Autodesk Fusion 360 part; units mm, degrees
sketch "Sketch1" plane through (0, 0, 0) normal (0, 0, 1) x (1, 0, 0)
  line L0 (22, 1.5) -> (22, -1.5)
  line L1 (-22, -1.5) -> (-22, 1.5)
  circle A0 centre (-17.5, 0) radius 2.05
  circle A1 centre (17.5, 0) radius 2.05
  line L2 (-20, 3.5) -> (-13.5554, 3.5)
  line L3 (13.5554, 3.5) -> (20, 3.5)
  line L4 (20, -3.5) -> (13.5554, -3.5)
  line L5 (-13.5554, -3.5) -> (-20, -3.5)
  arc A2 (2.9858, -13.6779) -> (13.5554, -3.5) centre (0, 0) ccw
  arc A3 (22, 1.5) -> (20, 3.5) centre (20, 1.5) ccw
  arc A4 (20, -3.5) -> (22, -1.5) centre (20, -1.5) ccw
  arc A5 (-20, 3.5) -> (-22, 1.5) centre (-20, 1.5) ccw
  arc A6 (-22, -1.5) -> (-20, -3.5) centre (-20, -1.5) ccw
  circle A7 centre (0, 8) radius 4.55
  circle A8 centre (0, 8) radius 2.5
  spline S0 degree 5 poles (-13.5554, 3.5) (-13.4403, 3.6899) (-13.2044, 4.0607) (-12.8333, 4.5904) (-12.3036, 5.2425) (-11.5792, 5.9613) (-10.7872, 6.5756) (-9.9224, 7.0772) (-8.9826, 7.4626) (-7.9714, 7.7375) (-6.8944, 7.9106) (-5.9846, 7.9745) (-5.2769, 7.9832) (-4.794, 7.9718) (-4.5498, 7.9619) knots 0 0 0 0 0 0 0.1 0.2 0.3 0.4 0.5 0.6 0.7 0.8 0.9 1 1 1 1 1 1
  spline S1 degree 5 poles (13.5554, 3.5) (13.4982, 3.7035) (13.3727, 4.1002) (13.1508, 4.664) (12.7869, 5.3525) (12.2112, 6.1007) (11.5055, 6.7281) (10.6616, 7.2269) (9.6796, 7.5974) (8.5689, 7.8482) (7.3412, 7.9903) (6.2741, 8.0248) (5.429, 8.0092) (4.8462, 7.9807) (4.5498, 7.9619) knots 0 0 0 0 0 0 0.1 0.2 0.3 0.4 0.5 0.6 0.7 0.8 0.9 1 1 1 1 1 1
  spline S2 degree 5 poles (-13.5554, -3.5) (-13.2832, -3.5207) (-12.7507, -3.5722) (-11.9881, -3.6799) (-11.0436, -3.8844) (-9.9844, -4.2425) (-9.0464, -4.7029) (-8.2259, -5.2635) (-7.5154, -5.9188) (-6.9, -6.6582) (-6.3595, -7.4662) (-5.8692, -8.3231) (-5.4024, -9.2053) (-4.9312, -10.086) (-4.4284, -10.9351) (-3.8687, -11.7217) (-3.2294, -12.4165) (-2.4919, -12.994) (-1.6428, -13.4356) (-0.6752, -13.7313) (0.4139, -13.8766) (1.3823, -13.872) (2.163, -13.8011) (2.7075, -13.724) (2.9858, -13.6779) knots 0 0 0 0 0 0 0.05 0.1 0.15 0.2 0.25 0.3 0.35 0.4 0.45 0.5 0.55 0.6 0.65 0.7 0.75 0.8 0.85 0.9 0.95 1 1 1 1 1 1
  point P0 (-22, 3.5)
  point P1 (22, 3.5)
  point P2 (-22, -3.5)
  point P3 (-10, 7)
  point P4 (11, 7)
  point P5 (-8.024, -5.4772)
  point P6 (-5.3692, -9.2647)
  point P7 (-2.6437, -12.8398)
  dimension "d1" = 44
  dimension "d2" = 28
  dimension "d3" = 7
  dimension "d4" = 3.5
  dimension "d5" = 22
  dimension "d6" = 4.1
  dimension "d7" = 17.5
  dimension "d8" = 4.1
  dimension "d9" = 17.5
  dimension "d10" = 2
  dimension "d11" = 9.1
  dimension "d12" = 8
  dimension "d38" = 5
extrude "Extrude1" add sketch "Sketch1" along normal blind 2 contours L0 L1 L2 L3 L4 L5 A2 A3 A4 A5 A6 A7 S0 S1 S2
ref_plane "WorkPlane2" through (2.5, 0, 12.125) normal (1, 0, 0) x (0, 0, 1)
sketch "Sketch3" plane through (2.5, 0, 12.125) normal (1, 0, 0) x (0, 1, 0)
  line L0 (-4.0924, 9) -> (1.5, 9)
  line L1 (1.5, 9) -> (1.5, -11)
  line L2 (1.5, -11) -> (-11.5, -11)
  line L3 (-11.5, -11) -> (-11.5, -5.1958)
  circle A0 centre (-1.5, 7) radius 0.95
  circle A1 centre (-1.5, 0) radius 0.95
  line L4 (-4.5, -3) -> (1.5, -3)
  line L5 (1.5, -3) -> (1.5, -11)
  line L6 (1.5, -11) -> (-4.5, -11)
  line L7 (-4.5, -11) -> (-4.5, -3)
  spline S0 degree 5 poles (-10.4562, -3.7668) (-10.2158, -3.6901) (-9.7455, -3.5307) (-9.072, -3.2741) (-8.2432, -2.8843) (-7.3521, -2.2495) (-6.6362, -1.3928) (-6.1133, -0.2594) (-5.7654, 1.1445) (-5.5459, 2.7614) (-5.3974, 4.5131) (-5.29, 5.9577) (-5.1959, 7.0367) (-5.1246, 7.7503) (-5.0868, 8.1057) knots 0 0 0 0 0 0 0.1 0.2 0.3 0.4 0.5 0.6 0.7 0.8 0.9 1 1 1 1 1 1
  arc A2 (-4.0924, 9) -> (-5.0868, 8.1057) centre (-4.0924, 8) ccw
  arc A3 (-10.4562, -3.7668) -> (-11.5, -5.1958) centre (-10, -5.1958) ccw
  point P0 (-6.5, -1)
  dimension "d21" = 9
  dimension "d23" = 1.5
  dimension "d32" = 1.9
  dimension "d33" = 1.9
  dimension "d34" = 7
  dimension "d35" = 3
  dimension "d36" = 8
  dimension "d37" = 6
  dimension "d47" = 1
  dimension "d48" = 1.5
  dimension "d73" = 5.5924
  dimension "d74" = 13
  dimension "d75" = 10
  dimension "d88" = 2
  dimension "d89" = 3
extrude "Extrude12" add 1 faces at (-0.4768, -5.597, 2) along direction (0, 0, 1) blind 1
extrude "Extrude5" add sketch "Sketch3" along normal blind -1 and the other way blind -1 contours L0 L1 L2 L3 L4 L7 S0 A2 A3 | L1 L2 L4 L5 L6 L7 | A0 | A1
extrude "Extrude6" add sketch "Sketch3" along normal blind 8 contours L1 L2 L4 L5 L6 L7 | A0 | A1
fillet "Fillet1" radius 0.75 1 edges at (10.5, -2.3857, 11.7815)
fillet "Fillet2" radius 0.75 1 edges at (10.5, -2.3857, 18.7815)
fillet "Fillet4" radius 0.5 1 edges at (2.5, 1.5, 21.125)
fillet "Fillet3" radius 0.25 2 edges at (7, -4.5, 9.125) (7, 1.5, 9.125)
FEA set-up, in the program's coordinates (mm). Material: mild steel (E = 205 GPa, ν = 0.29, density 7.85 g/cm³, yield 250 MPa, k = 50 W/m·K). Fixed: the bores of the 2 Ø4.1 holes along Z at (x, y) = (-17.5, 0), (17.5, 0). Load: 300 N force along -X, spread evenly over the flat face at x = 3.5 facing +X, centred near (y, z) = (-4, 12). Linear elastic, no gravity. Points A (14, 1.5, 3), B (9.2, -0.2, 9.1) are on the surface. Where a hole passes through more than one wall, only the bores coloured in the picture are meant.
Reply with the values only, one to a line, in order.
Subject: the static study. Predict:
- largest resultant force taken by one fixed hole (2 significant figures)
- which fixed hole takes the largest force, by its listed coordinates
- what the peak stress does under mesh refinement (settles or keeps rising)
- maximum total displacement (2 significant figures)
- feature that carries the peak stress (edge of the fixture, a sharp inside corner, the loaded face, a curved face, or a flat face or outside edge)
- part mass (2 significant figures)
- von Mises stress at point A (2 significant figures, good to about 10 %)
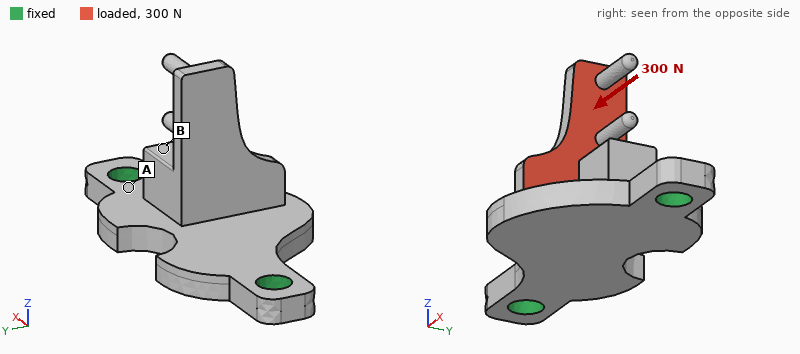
230 N
(17.5, 0)
keeps rising
76 µm
a sharp inside corner
17 g
33 MPa
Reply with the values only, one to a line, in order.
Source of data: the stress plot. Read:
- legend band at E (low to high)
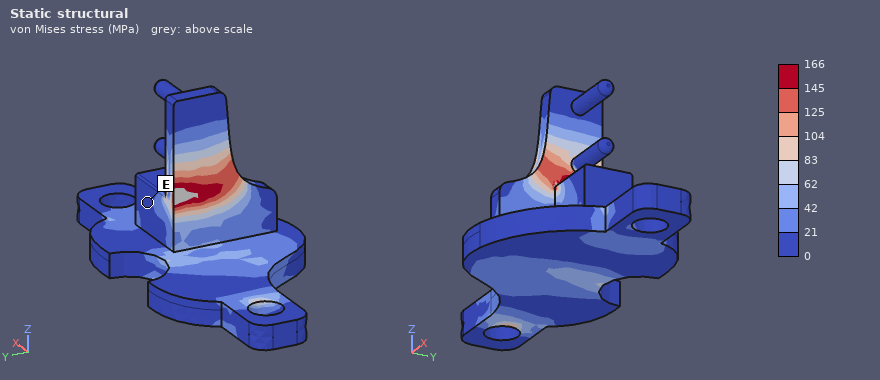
0 to 21 MPa
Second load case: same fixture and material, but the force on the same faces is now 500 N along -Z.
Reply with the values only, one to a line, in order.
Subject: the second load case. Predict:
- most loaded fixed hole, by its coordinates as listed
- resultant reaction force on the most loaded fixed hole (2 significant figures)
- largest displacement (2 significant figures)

(17.5, 0)
320 N
38 µm
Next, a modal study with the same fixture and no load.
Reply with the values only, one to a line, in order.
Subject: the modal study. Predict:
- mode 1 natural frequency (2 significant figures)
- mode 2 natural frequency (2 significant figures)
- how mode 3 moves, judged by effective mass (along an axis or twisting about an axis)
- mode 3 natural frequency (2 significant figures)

5900 Hz
7300 Hz
along Z
10 kHz
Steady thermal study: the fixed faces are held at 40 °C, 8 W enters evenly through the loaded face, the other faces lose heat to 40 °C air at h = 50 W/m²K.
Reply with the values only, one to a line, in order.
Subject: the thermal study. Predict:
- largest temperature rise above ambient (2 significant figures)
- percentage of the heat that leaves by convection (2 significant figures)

77 K
27 %
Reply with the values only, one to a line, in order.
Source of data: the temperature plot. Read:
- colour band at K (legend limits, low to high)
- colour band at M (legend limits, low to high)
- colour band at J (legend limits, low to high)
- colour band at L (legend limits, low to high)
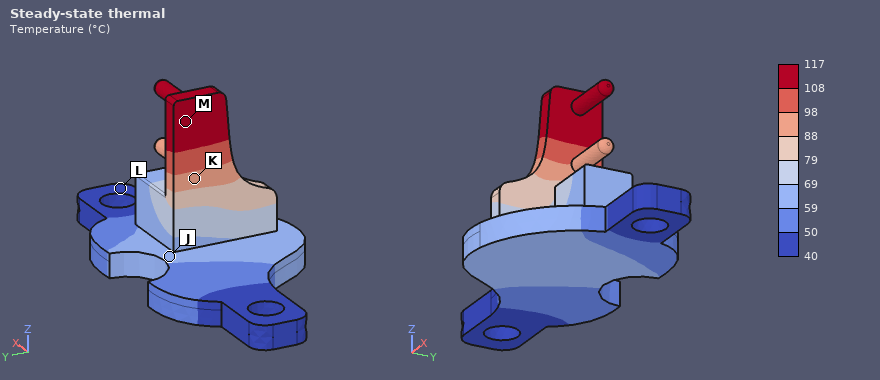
88 to 98 °C
108 to 117 °C
59 to 69 °C
40 to 50 °C
